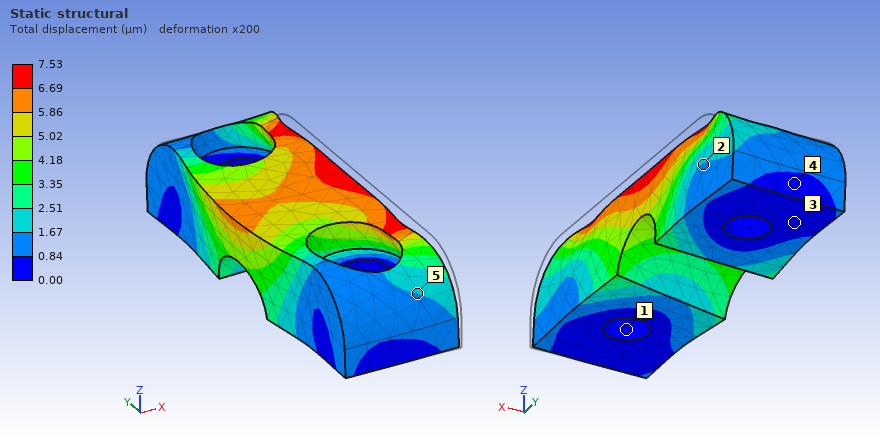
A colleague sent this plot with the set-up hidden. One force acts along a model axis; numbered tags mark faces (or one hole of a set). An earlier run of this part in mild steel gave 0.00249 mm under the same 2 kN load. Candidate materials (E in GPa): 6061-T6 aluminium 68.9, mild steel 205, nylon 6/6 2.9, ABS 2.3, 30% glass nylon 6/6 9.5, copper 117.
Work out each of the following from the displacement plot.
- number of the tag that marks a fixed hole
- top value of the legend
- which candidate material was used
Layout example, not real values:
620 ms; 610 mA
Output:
1; 7.53 µm; 6061-T6 aluminium
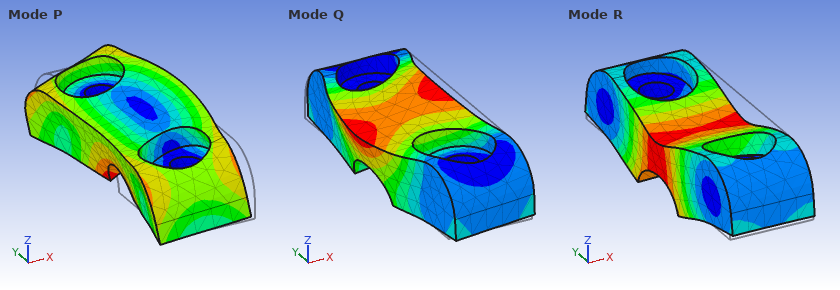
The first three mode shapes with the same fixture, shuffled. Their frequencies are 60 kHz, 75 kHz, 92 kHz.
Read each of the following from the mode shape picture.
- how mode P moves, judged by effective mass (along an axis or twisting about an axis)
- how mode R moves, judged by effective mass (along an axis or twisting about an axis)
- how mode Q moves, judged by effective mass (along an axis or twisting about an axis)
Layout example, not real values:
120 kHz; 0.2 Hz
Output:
twisting about Y; along Z; along X
